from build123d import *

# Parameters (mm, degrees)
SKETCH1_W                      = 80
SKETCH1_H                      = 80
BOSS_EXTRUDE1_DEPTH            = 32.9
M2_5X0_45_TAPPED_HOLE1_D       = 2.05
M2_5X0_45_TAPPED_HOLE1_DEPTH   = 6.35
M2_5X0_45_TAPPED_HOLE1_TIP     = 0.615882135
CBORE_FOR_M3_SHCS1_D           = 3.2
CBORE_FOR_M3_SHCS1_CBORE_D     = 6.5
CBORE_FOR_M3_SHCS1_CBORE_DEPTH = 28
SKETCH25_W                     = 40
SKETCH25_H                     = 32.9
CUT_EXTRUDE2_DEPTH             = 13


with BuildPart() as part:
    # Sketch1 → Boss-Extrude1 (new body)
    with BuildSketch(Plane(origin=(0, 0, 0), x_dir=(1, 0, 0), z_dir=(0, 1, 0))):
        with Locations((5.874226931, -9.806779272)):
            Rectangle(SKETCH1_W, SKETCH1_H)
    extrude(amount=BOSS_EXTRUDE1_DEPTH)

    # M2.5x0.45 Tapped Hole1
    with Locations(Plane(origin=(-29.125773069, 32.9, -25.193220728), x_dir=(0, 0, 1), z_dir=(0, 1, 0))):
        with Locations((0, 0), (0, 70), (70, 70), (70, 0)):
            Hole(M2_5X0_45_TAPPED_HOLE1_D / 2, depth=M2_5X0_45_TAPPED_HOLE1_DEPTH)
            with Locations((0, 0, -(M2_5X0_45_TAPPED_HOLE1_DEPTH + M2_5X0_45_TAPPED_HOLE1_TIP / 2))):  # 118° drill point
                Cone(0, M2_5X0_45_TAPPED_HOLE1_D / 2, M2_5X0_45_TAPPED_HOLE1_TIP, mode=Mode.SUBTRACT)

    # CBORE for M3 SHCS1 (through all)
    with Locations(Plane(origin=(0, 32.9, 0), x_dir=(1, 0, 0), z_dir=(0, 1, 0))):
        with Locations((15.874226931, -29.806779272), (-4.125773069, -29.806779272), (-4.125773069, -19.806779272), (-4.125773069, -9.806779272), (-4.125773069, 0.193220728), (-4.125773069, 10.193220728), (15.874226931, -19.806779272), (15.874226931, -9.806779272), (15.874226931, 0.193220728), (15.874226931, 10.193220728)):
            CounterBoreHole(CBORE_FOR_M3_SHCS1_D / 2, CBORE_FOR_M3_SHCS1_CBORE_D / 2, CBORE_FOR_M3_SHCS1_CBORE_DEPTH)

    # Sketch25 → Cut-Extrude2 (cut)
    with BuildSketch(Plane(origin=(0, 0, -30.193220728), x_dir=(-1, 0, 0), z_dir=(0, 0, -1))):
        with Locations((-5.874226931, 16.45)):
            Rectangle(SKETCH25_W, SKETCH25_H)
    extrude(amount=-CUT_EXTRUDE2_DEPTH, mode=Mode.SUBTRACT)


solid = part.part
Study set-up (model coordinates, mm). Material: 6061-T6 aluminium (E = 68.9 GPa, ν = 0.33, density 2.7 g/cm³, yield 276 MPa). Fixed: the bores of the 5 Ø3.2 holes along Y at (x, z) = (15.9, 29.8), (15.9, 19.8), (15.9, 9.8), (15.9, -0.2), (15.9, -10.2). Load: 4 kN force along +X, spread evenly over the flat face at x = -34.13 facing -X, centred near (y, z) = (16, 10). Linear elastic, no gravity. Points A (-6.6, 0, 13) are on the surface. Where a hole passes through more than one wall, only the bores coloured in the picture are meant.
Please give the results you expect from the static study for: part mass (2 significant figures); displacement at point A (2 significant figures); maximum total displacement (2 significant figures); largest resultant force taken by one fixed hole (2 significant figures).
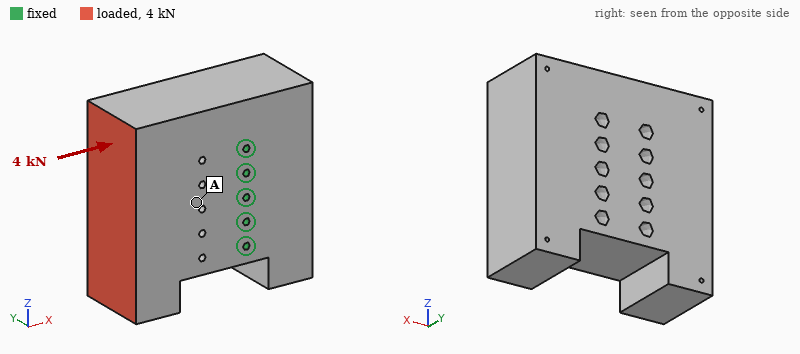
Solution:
500 g
0.055 mm
0.15 mm
900 N
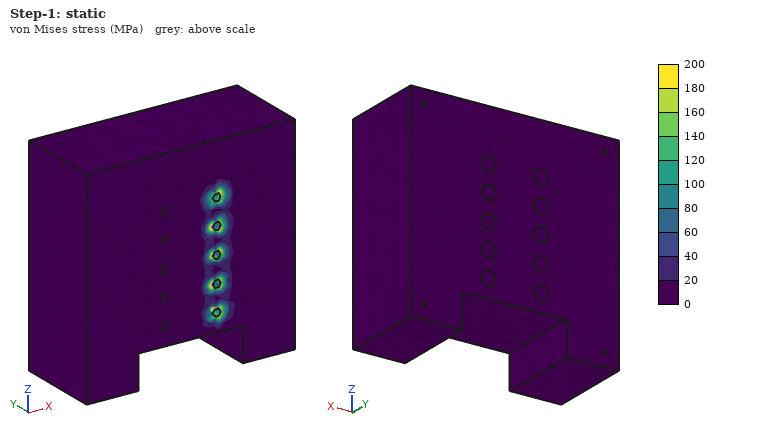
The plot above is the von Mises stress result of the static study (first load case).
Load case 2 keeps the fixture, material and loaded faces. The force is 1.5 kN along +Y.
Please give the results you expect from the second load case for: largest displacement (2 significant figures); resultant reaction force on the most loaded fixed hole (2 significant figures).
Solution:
0.20 mm
320 N
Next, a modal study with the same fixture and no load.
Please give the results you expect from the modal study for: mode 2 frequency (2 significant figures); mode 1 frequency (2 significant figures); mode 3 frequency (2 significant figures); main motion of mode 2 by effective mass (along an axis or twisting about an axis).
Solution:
4200 Hz
1100 Hz
4900 Hz
along Z
